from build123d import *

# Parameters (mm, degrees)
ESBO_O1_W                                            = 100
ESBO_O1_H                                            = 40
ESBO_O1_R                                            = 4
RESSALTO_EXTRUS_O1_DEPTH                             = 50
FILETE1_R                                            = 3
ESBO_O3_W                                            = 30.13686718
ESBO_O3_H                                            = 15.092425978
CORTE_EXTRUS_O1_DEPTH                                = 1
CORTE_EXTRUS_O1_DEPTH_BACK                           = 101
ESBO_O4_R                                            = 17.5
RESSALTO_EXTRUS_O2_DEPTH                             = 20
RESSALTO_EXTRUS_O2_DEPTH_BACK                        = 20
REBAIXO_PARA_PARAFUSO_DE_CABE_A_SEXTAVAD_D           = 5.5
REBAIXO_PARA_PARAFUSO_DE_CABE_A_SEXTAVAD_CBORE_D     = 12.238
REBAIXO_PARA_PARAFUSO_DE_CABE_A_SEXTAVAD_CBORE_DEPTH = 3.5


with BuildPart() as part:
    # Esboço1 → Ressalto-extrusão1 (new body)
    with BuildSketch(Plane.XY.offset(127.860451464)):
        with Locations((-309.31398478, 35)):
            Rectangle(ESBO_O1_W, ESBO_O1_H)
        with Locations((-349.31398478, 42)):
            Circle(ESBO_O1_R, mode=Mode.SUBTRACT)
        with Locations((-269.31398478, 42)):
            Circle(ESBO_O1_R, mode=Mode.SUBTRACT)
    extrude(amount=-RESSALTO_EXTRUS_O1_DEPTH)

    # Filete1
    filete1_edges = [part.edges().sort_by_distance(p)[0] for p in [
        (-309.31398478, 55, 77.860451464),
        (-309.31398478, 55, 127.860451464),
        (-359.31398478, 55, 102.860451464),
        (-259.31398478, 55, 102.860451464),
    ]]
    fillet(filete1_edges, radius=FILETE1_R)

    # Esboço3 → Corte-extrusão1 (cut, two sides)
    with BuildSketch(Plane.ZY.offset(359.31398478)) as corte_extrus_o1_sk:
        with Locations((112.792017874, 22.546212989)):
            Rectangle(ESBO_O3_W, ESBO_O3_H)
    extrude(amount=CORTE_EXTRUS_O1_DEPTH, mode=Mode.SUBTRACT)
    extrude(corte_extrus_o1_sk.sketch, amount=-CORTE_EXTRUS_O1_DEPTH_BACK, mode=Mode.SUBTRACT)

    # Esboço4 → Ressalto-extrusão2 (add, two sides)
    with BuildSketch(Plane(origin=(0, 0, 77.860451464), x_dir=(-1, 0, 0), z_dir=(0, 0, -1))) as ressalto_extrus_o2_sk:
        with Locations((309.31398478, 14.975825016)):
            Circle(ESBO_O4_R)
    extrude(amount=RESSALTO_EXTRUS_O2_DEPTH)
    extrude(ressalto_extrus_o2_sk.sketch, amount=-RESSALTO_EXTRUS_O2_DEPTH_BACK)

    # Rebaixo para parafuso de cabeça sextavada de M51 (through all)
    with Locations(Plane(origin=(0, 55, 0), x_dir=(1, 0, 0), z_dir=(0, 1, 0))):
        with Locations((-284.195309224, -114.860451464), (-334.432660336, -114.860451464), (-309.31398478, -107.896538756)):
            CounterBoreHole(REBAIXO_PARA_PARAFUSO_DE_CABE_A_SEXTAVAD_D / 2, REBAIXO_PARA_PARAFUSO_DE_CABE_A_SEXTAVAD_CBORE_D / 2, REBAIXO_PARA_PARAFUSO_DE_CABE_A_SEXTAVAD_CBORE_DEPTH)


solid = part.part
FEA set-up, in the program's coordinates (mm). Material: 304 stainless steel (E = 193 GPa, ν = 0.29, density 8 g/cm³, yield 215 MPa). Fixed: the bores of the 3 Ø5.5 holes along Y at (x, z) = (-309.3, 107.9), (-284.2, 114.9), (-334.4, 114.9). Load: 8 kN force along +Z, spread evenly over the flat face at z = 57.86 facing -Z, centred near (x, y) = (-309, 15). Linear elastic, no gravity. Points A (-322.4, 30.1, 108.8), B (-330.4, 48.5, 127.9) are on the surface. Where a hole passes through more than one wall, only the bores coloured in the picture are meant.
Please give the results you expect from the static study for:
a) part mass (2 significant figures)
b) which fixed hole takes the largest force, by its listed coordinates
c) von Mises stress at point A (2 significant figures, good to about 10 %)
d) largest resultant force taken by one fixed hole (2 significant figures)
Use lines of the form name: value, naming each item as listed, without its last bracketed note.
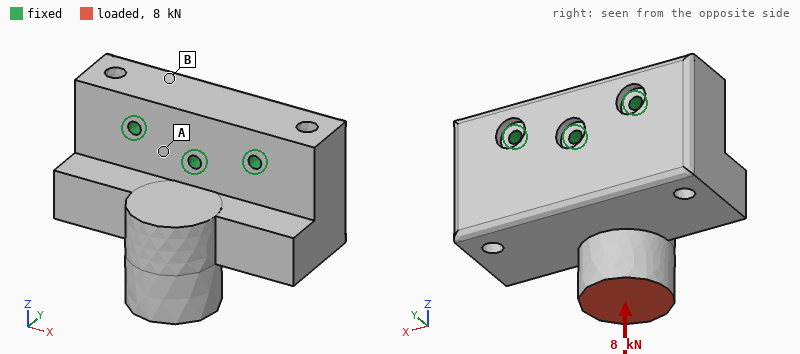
part mass: 1.4 kg
which fixed hole takes the largest force, by its listed coordinates: (-309.3, 107.9)
von Mises stress at point A: 17 MPa
largest resultant force taken by one fixed hole: 4.2 kN
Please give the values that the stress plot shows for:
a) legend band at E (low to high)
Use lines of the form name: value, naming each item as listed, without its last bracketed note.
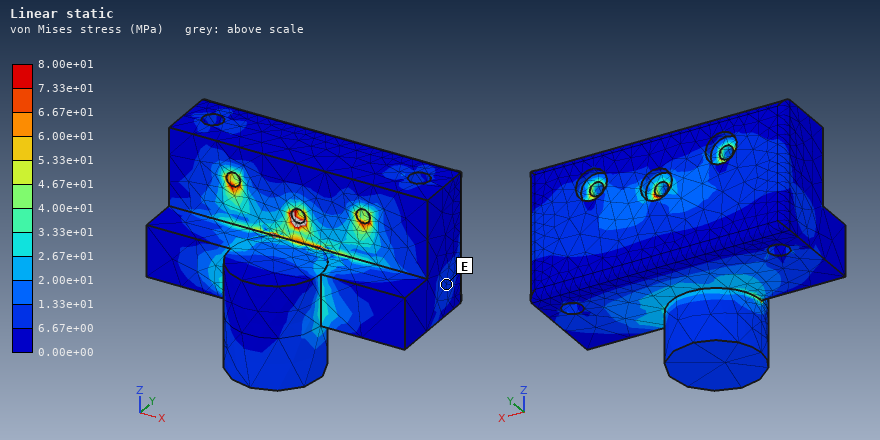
legend band at E: 6.67e+00 to 1.33e+01 MPa
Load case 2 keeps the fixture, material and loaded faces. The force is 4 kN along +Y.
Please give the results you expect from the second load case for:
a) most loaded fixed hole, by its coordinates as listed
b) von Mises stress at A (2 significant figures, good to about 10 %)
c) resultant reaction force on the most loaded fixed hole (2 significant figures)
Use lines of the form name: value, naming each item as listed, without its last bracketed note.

most loaded fixed hole, by its coordinates as listed: (-309.3, 107.9)
von Mises stress at A: 14 MPa
resultant reaction force on the most loaded fixed hole: 3.7 kN
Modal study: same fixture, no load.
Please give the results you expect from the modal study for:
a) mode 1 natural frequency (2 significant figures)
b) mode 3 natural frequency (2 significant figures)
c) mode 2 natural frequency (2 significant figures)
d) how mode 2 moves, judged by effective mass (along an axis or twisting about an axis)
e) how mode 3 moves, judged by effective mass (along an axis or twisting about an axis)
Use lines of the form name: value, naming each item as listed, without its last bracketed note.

mode 1 natural frequency: 4200 Hz
mode 3 natural frequency: 8800 Hz
mode 2 natural frequency: 6700 Hz
how mode 2 moves, judged by effective mass: along X
how mode 3 moves, judged by effective mass: along X
